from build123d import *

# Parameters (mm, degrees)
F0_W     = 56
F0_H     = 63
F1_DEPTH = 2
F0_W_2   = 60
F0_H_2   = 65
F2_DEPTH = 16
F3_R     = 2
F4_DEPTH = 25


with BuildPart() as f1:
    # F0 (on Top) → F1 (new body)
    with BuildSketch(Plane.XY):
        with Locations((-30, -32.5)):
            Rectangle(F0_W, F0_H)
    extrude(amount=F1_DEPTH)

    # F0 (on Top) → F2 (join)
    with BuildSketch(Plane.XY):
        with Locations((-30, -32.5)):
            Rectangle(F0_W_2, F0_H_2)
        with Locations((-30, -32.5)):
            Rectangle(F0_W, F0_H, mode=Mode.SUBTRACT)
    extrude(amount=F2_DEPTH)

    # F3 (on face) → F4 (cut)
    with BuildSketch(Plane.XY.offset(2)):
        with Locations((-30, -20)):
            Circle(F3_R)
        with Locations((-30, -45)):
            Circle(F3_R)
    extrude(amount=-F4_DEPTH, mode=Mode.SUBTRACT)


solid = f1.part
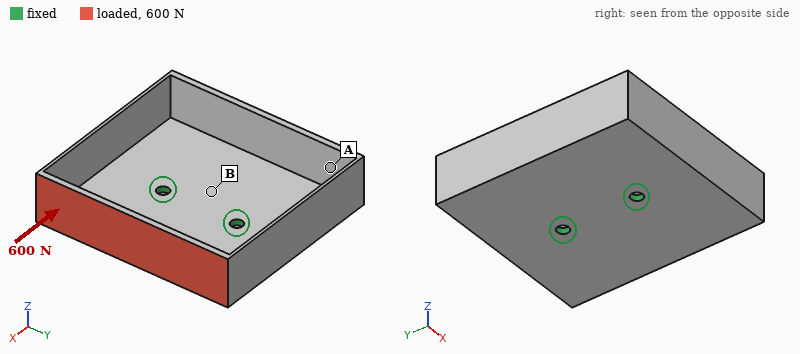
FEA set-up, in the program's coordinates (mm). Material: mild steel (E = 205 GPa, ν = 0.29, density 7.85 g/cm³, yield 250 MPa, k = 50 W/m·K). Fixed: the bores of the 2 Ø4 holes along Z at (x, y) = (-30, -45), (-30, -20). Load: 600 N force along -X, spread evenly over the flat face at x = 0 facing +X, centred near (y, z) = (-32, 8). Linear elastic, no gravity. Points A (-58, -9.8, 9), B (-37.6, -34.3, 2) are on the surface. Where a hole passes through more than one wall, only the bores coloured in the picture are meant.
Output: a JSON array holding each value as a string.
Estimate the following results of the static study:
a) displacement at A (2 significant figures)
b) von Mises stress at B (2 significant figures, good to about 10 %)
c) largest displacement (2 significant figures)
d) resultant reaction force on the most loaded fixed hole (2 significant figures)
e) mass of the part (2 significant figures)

["0.075 mm", "32 MPa", "0.15 mm", "310 N", "100 g"]
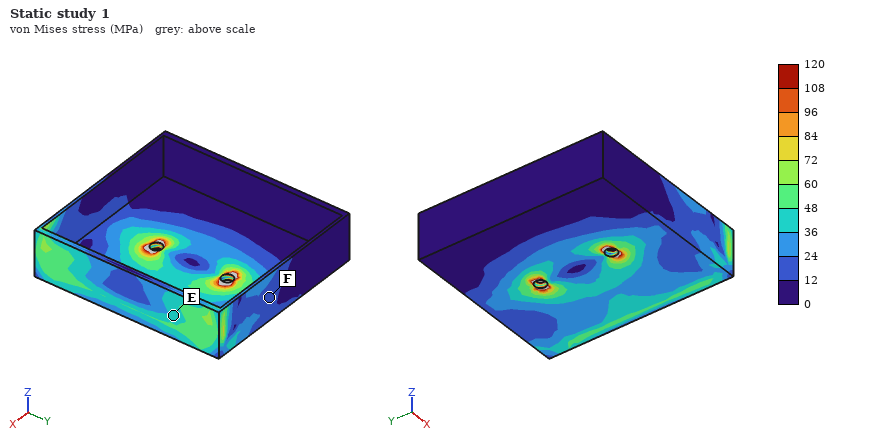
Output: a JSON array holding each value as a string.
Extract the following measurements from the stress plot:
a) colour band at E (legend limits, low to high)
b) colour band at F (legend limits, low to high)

["36 to 48 MPa", "12 to 24 MPa"]
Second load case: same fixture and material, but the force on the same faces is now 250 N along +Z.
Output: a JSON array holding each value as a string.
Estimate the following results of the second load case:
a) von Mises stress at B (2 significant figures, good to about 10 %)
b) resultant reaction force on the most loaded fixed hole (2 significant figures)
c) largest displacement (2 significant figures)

["41 MPa", "130 N", "0.20 mm"]
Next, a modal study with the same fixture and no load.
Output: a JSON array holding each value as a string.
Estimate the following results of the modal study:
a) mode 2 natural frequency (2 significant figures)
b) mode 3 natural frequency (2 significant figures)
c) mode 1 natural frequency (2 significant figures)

["1400 Hz", "1700 Hz", "940 Hz"]
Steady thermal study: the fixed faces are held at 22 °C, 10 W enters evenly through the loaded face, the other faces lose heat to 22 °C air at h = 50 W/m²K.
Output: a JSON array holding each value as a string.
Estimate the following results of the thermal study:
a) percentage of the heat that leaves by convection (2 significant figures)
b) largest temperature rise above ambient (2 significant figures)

["62 %", "34 K"]
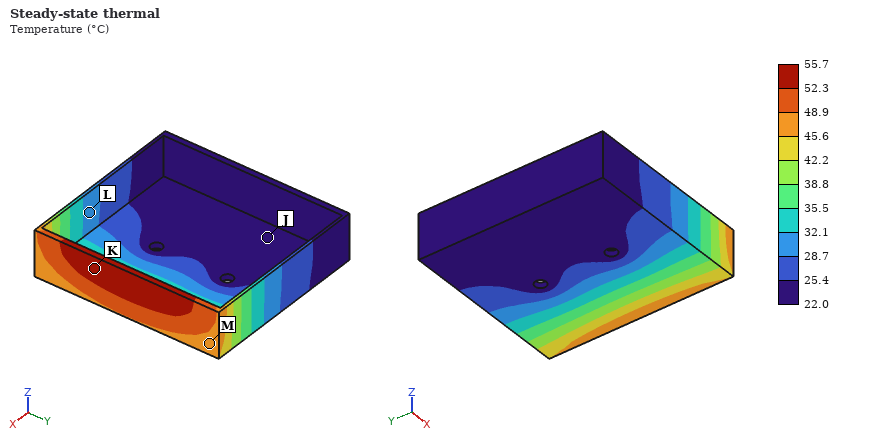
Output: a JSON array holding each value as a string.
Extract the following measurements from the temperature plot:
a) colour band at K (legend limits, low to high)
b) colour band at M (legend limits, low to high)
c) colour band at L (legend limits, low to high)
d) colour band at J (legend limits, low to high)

["52.3 to 55.7 °C", "45.6 to 48.9 °C", "28.7 to 32.1 °C", "22.0 to 25.4 °C"]
